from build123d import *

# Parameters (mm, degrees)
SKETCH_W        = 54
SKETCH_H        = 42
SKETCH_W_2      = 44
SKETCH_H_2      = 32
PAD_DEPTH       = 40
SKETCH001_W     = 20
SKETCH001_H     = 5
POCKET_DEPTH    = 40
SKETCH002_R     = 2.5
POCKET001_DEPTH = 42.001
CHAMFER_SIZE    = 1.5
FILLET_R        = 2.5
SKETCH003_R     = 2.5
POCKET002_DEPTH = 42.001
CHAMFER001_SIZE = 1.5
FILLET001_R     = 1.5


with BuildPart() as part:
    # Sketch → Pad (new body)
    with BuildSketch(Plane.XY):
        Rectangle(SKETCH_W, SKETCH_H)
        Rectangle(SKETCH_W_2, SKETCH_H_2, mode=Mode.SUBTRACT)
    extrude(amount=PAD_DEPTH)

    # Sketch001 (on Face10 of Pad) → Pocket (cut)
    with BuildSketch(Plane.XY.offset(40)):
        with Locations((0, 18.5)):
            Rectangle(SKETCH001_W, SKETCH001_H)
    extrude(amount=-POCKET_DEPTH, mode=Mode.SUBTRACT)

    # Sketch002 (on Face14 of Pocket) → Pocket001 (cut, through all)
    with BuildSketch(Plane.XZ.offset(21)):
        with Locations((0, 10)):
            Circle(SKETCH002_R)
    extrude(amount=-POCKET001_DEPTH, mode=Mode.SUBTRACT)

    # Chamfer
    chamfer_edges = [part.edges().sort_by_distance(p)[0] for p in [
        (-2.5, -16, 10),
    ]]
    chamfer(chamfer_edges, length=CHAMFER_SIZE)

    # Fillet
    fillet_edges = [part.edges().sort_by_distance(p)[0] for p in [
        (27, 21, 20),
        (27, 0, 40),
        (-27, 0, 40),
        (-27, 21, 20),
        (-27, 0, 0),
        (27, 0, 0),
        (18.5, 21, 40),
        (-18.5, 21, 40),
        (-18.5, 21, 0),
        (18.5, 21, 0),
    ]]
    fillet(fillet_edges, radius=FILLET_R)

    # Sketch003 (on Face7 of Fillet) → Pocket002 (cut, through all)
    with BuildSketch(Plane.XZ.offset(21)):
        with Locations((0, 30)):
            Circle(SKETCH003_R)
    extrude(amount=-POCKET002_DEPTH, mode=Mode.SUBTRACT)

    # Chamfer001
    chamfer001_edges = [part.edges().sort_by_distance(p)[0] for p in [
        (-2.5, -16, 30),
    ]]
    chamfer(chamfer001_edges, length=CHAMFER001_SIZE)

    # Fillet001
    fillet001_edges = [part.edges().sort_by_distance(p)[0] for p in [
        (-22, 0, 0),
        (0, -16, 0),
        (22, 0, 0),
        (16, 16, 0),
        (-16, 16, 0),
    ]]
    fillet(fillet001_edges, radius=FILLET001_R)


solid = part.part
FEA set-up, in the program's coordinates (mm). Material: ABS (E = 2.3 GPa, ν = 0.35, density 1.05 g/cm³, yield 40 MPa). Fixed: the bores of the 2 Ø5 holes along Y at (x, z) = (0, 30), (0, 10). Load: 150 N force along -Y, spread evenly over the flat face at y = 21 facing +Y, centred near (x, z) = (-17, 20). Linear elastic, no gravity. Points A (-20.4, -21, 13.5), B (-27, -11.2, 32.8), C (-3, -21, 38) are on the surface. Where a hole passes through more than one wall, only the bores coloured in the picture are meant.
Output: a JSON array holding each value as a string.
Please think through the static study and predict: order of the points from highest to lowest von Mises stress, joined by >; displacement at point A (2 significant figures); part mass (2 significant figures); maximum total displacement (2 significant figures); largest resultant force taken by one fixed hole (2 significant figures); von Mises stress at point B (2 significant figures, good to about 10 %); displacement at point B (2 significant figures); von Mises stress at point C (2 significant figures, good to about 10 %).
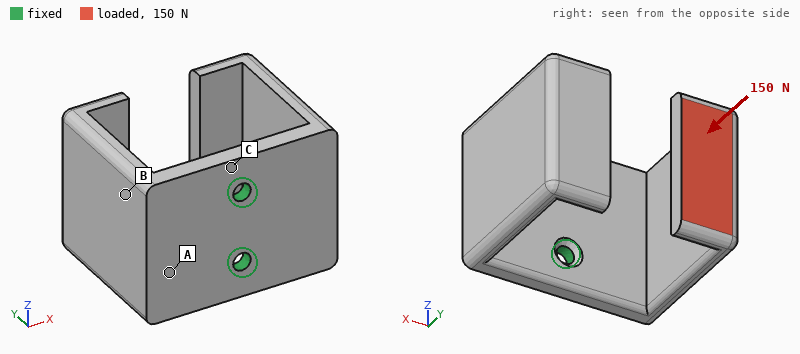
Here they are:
["C > B > A", "0.41 mm", "31 g", "0.81 mm", "76 N", "5.6 MPa", "0.56 mm", "8.3 MPa"]
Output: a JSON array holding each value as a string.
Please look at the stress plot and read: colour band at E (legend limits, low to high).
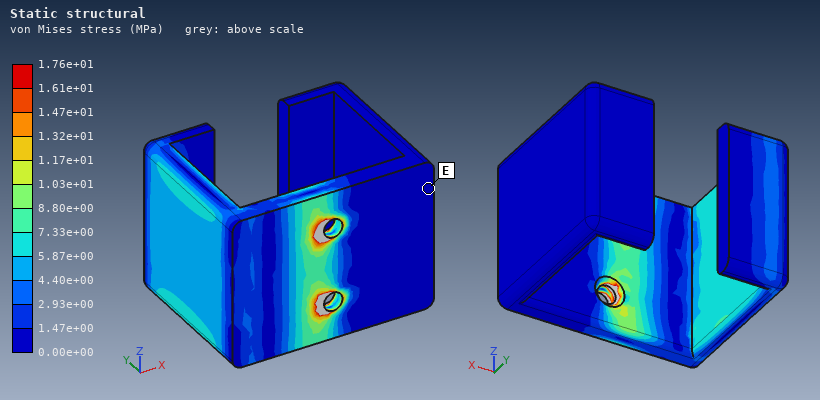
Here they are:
["0.00e+00 to 1.47e+00 MPa"]
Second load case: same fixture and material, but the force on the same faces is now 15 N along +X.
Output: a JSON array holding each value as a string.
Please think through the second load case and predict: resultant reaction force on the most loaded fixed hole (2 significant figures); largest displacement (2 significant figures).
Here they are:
["7.7 N", "0.89 mm"]
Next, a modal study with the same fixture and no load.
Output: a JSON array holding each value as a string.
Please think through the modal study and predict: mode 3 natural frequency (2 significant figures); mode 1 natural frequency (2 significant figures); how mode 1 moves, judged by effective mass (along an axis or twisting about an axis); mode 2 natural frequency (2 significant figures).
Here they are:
["490 Hz", "280 Hz", "along X", "300 Hz"]
